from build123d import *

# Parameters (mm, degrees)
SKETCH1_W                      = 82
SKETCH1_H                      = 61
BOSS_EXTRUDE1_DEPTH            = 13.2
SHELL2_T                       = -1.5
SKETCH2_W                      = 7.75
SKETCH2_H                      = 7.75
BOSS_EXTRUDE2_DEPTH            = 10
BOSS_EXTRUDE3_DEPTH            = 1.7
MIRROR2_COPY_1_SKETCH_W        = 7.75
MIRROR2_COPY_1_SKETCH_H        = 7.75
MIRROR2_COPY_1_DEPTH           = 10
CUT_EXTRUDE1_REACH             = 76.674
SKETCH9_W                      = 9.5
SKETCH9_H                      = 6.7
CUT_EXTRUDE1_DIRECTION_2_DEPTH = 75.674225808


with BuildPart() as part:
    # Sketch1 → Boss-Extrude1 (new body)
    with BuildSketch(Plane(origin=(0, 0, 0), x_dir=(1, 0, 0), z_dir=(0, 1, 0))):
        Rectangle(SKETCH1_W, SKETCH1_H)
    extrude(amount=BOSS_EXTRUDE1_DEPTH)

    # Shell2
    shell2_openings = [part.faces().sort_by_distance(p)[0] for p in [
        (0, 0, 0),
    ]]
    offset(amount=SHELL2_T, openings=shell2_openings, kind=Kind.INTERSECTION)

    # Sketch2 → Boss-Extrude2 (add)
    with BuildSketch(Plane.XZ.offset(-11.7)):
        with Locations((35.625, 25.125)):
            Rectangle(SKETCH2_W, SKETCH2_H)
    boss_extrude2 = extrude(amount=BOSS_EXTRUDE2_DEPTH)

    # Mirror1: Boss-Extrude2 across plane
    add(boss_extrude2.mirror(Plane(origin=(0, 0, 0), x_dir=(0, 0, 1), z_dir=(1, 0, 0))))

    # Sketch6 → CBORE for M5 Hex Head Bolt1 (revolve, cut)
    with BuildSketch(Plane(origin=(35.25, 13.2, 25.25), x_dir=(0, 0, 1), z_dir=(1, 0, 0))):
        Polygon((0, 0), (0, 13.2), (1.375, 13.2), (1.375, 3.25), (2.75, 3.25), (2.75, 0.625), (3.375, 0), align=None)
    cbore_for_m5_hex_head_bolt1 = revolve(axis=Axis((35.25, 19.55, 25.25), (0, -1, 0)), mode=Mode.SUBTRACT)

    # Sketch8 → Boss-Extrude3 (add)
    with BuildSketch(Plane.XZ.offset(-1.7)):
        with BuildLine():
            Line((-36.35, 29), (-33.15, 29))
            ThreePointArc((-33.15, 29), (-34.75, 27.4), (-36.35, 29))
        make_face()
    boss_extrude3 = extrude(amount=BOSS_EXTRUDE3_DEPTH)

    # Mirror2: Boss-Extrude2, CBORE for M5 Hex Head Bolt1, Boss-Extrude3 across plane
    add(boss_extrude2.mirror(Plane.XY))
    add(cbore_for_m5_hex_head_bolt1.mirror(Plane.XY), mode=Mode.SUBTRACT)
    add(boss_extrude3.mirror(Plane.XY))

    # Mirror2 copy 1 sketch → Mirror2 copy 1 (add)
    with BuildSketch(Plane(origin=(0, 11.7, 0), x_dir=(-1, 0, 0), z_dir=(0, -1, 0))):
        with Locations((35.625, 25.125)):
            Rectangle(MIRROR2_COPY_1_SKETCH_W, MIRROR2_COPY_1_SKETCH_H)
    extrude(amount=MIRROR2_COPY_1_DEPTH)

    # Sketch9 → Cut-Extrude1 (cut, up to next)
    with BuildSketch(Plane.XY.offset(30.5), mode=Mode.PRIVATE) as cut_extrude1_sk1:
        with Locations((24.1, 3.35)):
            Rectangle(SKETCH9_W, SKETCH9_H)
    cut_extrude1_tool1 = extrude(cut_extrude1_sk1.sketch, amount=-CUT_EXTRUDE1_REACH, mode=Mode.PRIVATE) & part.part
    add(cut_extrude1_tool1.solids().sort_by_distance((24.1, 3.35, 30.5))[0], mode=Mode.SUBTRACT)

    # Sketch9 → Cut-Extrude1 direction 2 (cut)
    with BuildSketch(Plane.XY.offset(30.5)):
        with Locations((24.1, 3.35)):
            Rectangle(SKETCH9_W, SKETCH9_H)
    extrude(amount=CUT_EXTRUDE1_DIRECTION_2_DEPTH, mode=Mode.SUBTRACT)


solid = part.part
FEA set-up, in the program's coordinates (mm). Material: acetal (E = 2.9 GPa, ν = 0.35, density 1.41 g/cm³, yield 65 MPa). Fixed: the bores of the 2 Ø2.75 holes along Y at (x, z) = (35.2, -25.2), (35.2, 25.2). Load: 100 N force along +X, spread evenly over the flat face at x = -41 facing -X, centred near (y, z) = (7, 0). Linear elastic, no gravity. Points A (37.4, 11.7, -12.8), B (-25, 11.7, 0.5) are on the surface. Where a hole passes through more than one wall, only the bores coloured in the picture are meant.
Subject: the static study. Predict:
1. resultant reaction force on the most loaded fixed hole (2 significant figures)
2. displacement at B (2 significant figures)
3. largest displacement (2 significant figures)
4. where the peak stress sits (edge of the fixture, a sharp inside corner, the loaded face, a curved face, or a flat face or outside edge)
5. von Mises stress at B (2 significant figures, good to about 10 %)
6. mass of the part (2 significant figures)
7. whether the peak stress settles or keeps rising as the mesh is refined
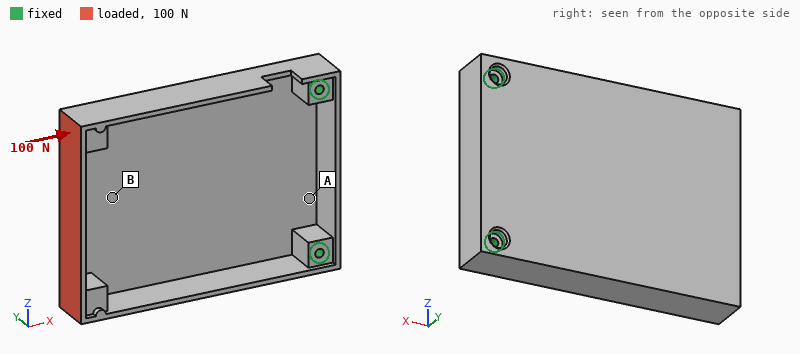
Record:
51 N
0.41 mm
1.2 mm
a sharp inside corner
3.2 MPa
20 g
keeps rising
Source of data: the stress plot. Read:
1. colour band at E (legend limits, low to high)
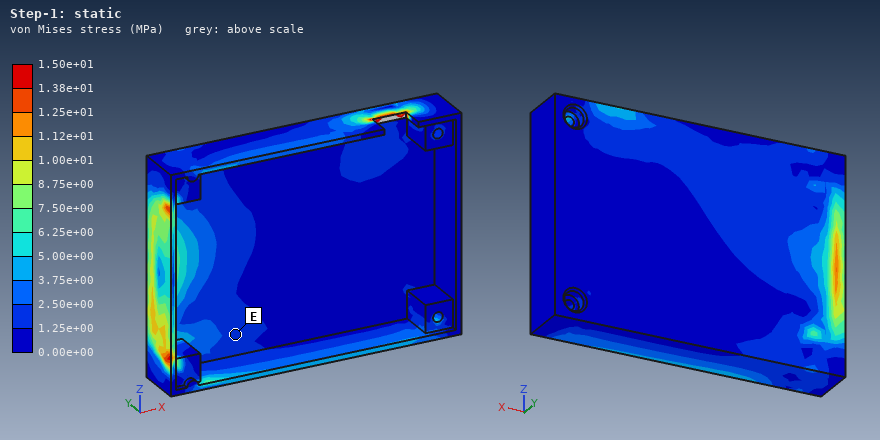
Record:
1.25e+00 to 2.50e+00 MPa
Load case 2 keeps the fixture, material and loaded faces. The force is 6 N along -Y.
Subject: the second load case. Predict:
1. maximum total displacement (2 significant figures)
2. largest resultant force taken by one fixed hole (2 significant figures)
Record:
1.0 mm
3.1 N
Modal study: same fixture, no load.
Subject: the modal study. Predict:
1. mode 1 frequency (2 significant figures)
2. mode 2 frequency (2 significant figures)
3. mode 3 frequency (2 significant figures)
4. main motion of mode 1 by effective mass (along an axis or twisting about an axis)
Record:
170 Hz
320 Hz
650 Hz
along Y
